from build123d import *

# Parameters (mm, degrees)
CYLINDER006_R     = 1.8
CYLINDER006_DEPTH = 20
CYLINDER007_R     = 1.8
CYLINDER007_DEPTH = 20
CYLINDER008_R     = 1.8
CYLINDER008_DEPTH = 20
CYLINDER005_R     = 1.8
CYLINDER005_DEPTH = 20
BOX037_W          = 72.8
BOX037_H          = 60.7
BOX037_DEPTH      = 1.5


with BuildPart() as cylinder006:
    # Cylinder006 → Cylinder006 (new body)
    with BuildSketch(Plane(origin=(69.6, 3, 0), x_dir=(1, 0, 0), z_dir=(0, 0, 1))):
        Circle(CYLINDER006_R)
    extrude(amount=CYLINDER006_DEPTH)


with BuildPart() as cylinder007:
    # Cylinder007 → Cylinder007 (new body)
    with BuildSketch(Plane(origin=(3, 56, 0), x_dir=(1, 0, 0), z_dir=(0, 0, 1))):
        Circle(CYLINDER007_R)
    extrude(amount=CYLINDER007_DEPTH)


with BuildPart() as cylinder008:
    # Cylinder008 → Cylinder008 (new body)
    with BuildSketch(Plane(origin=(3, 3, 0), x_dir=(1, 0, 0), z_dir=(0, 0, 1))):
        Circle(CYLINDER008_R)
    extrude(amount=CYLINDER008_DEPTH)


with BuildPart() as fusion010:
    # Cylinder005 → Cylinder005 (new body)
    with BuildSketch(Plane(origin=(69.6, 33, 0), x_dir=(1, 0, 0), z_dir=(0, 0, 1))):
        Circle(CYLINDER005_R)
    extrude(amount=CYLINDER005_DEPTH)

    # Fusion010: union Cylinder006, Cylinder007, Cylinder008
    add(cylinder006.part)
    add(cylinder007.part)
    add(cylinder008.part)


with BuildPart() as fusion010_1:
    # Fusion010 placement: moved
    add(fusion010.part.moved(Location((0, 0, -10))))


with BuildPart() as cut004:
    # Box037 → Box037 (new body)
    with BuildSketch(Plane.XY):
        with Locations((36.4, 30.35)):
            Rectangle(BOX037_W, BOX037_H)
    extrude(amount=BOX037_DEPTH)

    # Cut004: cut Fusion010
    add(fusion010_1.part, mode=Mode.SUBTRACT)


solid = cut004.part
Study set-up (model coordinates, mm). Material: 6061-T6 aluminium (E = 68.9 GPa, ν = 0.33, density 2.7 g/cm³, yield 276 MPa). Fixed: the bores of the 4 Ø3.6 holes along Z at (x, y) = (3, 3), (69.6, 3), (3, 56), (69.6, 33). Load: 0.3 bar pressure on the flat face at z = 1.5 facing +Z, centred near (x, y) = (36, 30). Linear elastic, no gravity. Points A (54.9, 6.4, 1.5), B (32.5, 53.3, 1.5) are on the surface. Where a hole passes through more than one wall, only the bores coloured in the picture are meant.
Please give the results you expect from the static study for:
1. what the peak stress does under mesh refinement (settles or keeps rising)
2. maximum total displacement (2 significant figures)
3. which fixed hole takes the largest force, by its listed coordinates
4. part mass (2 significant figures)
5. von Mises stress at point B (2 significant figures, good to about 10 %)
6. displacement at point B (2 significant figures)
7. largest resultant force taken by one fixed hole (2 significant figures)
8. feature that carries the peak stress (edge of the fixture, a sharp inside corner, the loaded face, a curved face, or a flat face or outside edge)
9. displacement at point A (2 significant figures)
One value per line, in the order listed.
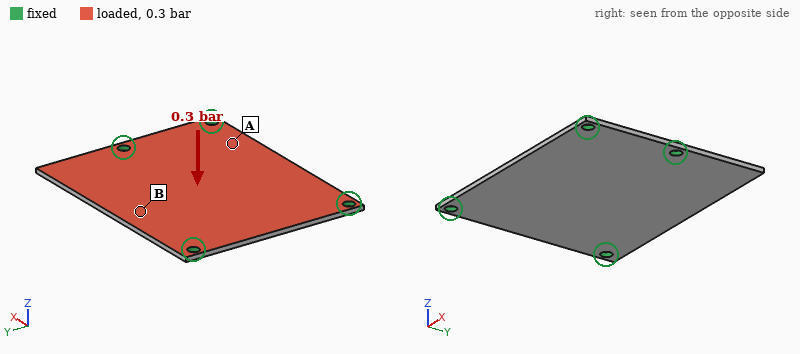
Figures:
keeps rising
0.18 mm
(69.6, 33)
18 g
20 MPa
0.14 mm
50 N
edge of the fixture
0.044 mm
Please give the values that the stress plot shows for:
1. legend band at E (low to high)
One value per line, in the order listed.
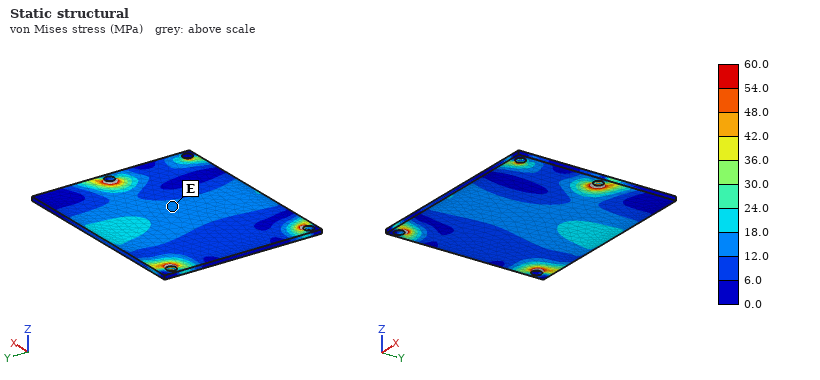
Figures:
12.0 to 18.0 MPa
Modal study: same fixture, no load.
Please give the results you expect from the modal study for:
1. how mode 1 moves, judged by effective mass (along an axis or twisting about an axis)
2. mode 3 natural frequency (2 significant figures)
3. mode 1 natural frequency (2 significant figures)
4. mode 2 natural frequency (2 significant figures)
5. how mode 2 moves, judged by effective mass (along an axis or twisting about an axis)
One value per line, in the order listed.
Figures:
along Z
2600 Hz
1300 Hz
1700 Hz
along Z
